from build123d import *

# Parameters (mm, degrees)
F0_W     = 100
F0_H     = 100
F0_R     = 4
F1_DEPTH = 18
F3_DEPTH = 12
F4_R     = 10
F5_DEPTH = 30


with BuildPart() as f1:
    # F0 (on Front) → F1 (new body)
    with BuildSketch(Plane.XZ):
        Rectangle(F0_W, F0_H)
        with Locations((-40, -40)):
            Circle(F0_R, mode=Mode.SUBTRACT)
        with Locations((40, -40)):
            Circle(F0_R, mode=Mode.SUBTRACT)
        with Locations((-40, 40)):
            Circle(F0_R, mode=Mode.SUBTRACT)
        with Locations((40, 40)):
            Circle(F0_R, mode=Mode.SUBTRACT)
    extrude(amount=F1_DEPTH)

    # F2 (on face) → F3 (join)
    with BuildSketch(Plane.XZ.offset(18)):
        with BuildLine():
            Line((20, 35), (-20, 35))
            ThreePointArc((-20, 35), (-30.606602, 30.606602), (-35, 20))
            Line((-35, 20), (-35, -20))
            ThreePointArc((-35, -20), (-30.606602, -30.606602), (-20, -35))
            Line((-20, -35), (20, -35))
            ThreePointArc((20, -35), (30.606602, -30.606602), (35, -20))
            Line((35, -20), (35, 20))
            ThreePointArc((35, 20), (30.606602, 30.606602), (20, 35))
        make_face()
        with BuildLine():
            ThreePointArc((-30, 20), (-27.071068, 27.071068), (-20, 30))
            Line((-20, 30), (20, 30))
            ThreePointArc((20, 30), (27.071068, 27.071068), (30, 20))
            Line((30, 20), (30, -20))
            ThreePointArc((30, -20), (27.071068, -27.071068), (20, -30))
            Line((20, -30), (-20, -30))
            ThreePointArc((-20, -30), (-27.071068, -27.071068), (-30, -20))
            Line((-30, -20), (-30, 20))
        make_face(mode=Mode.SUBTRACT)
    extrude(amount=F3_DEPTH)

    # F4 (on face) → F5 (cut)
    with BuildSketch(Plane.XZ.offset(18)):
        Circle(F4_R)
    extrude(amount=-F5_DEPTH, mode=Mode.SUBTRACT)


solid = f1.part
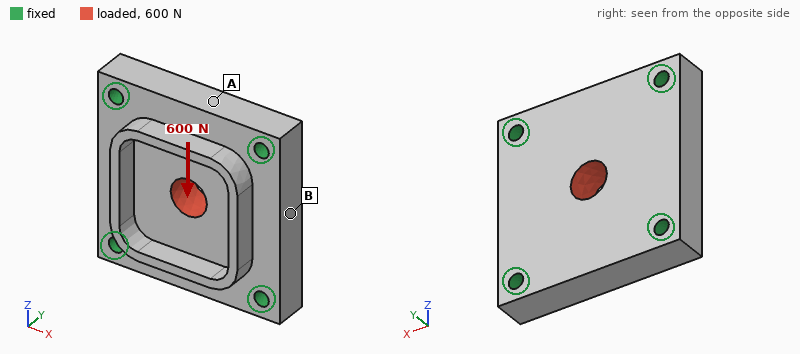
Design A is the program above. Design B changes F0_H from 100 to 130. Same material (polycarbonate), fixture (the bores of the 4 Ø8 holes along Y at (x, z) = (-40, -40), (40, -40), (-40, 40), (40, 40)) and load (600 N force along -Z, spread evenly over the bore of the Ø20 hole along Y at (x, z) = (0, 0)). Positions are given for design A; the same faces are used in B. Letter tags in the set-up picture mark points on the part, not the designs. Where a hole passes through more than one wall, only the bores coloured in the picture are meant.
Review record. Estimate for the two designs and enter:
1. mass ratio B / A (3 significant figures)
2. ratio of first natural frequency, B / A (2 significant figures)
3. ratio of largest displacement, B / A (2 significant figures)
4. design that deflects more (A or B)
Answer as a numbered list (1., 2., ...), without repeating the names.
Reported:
1. 1.29
2. 1.0
3. 0.88
4. A
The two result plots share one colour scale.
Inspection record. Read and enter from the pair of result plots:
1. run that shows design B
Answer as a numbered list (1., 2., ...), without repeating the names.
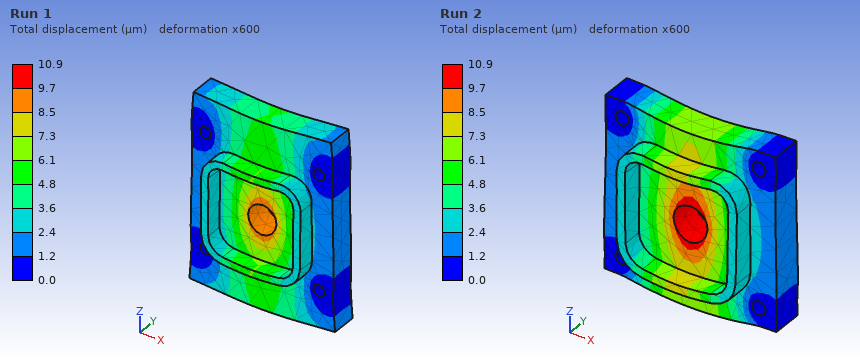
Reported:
1. Run 1
